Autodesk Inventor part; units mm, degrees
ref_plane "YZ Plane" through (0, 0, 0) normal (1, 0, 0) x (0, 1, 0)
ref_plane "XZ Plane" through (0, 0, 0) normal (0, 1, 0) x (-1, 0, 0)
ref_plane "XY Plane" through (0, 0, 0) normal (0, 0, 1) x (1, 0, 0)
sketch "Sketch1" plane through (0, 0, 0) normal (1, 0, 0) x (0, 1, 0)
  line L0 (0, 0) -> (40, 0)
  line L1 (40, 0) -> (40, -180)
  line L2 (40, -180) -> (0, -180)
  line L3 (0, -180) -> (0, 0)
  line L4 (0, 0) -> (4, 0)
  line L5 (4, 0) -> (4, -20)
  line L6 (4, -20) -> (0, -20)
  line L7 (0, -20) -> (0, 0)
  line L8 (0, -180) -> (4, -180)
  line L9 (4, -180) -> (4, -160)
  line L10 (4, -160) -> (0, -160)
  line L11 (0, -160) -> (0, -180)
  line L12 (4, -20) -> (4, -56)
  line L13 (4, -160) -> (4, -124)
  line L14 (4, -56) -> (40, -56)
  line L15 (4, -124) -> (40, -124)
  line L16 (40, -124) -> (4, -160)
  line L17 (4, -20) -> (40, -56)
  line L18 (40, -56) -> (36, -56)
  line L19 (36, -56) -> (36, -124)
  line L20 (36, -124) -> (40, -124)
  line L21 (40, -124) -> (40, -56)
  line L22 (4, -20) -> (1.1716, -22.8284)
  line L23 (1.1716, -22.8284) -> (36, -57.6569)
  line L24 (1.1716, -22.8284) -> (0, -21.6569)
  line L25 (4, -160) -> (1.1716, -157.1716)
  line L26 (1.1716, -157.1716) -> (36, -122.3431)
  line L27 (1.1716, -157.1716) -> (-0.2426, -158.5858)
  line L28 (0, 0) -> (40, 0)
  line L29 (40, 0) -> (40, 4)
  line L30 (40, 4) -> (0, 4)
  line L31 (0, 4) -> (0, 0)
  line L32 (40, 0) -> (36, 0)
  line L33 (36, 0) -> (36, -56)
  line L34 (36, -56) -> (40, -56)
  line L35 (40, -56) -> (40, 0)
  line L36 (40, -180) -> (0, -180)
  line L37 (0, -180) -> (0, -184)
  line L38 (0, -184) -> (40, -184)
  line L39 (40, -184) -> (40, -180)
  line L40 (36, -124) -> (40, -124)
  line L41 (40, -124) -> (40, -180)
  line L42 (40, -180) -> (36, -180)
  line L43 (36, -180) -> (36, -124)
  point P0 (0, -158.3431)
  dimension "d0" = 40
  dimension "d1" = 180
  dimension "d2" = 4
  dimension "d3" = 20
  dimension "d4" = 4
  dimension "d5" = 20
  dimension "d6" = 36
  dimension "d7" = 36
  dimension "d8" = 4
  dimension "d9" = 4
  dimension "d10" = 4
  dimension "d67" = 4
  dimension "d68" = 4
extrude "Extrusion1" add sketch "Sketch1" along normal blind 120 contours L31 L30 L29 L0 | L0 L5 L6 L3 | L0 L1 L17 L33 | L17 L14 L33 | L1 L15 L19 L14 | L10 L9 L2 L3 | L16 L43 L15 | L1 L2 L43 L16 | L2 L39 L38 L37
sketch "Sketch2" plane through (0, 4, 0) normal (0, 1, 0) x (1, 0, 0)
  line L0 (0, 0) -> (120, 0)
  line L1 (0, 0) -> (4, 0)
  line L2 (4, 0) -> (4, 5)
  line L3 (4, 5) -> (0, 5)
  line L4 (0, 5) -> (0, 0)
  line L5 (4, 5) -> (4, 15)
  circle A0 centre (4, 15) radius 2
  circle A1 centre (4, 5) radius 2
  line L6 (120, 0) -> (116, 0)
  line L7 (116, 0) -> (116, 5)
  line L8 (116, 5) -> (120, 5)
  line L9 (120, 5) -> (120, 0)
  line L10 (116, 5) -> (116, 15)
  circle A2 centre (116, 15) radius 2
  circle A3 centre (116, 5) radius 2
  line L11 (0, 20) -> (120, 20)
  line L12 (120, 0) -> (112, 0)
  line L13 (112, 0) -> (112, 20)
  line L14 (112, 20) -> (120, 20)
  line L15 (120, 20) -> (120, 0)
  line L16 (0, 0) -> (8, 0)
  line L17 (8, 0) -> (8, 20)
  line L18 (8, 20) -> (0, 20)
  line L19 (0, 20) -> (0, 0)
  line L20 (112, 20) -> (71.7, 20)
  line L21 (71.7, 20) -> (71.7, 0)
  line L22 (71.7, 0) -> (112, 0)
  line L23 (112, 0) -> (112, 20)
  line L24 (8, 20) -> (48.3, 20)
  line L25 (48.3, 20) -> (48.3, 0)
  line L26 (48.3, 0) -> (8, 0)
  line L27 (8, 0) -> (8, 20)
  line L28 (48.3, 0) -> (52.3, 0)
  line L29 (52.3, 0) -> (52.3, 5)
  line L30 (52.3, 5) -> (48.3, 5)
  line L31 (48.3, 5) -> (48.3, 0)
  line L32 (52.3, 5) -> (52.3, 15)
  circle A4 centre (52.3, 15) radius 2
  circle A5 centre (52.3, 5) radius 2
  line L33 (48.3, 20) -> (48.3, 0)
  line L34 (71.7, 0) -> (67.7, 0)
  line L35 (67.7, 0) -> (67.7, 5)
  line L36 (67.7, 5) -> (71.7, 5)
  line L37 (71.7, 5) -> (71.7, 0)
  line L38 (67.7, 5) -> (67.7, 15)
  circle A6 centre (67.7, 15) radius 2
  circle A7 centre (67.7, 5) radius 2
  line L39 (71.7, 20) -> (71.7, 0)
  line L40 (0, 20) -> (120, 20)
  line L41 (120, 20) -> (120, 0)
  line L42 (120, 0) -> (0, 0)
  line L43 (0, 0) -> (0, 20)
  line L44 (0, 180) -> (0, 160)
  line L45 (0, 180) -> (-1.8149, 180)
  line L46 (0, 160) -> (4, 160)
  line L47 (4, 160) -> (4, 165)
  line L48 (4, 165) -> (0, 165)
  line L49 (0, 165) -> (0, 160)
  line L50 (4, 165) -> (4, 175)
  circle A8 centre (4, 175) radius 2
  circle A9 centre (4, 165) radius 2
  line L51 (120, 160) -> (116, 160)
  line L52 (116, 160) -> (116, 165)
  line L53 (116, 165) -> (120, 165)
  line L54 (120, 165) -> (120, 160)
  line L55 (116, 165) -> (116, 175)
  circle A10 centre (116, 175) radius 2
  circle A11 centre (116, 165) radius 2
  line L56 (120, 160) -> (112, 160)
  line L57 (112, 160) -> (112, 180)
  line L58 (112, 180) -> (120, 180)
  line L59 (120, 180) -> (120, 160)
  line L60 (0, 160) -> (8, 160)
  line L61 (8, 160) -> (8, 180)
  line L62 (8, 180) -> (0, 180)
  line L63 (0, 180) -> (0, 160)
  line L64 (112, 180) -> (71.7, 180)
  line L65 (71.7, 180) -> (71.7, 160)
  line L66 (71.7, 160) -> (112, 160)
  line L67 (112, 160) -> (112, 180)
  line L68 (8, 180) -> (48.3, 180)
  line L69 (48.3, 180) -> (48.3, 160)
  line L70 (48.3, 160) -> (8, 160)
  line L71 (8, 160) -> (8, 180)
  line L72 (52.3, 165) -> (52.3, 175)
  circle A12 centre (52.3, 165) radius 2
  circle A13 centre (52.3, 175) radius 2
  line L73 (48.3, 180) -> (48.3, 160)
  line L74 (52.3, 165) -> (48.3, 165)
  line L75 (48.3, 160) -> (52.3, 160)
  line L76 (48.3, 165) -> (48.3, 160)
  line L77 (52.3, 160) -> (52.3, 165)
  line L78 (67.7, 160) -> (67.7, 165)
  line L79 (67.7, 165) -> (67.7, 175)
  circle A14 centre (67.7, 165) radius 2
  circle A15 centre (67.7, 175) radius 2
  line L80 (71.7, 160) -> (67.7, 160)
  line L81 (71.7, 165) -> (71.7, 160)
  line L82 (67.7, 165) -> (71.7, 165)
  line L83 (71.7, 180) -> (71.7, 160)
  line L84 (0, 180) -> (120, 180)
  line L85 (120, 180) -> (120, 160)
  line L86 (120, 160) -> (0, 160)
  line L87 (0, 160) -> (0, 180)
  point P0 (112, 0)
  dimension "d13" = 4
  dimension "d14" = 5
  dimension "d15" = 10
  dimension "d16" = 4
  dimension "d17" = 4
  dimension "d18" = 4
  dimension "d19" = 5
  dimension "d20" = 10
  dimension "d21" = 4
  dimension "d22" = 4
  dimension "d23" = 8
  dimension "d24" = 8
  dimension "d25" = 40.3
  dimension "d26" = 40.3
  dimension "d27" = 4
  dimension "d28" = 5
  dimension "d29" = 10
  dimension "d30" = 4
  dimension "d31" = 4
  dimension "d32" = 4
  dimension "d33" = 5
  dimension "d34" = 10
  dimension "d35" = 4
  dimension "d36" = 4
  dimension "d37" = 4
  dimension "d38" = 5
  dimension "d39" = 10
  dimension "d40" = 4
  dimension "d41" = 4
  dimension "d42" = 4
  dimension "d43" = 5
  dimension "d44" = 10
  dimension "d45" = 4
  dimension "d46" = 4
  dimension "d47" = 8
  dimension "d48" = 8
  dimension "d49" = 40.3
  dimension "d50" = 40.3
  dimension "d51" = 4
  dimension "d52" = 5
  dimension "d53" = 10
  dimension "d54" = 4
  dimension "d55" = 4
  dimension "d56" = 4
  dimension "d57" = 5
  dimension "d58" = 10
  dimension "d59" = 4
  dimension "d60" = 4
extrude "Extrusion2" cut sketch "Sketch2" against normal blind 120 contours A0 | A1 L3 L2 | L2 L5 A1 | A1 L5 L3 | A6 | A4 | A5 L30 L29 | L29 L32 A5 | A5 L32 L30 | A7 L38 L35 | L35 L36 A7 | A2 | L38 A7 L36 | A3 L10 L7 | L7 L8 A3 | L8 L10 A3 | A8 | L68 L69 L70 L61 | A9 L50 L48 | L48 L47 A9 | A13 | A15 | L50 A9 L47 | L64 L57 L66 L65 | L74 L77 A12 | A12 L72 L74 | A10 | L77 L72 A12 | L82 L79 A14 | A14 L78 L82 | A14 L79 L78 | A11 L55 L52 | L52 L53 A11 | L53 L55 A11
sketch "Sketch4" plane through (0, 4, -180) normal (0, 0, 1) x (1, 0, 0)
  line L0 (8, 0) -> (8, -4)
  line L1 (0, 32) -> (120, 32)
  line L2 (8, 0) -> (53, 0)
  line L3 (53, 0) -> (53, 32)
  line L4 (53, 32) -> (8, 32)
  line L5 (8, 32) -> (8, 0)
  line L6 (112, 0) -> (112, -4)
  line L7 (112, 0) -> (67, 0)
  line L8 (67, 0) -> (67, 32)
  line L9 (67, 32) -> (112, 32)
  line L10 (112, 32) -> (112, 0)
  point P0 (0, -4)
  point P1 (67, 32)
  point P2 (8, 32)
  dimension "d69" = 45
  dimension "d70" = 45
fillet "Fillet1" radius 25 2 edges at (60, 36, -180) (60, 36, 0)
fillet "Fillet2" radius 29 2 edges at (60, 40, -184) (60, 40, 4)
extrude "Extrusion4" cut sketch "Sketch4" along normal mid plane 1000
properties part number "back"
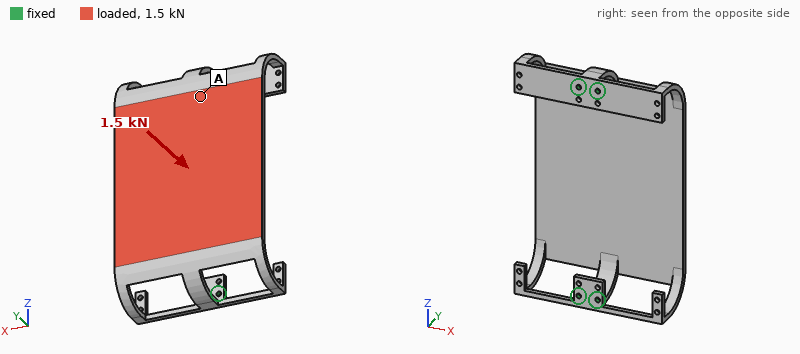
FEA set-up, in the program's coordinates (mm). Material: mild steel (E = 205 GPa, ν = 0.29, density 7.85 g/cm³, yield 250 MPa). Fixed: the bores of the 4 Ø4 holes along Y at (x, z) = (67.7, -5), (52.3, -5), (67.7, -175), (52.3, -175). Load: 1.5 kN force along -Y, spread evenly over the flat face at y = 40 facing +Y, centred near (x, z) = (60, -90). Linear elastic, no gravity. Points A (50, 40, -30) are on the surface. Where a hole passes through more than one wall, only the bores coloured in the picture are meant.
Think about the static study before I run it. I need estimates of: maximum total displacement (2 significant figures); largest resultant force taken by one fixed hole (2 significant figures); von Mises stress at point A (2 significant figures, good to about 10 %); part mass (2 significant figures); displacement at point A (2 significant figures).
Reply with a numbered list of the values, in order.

1. 0.52 mm
2. 580 N
3. 35 MPa
4. 760 g
5. 0.18 mm
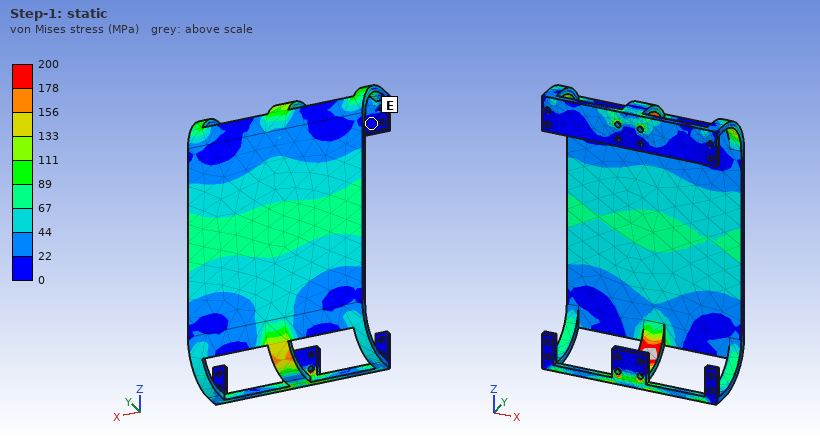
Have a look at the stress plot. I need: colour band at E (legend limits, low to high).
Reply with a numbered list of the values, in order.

1. 0 to 22 MPa
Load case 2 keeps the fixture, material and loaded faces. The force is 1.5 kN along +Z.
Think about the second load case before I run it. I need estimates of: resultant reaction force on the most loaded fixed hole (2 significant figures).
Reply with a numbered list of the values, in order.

1. 470 N
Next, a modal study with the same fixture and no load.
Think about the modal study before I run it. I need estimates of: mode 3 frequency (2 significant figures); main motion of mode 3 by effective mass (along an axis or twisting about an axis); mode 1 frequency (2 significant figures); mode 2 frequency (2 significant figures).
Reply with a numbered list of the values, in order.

1. 510 Hz
2. along Z
3. 430 Hz
4. 440 Hz
